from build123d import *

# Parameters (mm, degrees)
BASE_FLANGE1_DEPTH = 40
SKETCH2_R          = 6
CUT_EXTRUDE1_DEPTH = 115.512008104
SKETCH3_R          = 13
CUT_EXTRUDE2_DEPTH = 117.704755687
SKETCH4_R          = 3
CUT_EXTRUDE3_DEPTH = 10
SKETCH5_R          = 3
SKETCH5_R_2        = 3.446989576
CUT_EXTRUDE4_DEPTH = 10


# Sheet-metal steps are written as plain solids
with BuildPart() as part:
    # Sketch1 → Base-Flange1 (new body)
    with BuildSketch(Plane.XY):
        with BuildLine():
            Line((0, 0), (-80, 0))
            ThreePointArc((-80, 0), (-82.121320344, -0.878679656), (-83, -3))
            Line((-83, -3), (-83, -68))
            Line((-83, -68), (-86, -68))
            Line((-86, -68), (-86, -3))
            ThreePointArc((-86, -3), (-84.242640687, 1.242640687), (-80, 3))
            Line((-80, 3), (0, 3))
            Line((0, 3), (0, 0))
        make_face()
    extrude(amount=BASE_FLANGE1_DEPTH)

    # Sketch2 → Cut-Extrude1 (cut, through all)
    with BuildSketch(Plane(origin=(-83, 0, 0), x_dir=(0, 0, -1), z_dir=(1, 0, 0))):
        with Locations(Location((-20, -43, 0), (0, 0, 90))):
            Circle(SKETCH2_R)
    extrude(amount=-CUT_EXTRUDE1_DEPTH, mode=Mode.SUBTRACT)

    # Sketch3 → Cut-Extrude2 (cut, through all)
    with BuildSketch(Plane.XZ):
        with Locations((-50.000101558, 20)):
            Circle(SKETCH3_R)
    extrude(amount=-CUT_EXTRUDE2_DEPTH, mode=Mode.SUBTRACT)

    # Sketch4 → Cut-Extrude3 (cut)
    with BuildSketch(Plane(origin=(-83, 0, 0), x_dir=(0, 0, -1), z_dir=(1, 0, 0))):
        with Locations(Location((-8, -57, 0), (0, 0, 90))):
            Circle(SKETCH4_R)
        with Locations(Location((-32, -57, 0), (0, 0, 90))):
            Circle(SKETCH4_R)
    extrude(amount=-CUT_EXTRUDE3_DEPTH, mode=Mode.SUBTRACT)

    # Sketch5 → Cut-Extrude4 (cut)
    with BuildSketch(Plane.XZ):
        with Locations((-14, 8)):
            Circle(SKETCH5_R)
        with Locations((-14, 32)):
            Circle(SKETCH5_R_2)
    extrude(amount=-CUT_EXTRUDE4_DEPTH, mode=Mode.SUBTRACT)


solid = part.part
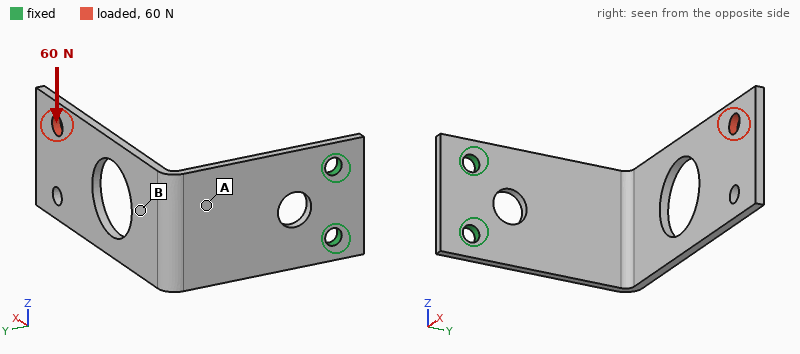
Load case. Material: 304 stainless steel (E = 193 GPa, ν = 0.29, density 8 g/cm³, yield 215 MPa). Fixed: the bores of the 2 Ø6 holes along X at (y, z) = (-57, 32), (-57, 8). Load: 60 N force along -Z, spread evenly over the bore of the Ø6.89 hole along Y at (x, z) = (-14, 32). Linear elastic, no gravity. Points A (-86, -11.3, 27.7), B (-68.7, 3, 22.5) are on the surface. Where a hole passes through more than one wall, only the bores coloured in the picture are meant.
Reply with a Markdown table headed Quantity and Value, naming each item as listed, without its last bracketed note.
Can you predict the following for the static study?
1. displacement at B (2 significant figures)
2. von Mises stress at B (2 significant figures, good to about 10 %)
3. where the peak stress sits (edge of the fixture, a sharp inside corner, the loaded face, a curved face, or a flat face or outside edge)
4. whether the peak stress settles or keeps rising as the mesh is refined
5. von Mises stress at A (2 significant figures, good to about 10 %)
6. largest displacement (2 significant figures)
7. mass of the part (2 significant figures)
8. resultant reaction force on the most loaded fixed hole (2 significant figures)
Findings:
| Quantity | Value |
|---|---|
| displacement at B | 0.12 mm |
| von Mises stress at B | 7.1 MPa |
| where the peak stress sits | edge of the fixture |
| whether the peak stress settles or keeps rising as the mesh is refined | keeps rising |
| von Mises stress at A | 54 MPa |
| largest displacement | 0.65 mm |
| mass of the part | 130 g |
| resultant reaction force on the most loaded fixed hole | 180 N |
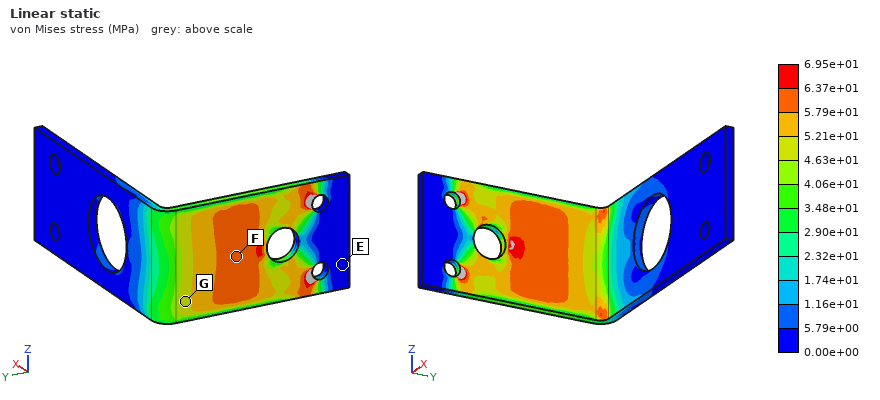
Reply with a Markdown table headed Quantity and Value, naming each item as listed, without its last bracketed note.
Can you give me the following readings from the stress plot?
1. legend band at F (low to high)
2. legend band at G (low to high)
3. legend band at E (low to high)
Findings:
| Quantity | Value |
|---|---|
| legend band at F | 5.79e+01 to 6.37e+01 MPa |
| legend band at G | 4.63e+01 to 5.21e+01 MPa |
| legend band at E | 0.00e+00 to 5.79e+00 MPa |
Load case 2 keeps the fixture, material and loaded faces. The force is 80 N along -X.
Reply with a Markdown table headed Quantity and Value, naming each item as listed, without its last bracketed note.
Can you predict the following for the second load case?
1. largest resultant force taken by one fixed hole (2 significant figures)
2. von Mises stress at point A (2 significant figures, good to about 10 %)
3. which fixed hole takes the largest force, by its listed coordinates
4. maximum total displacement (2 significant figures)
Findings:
| Quantity | Value |
|---|---|
| largest resultant force taken by one fixed hole | 70 N |
| von Mises stress at point A | 22 MPa |
| which fixed hole takes the largest force, by its listed coordinates | (-57, 32) |
| maximum total displacement | 0.82 mm |
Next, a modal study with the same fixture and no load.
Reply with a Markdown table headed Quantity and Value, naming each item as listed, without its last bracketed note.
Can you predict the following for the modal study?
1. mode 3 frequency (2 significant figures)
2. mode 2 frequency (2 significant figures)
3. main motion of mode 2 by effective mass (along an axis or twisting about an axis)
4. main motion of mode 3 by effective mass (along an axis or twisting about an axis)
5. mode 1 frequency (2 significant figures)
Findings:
| Quantity | Value |
|---|---|
| mode 3 frequency | 440 Hz |
| mode 2 frequency | 280 Hz |
| main motion of mode 2 by effective mass | along Z |
| main motion of mode 3 by effective mass | along X |
| mode 1 frequency | 150 Hz |
